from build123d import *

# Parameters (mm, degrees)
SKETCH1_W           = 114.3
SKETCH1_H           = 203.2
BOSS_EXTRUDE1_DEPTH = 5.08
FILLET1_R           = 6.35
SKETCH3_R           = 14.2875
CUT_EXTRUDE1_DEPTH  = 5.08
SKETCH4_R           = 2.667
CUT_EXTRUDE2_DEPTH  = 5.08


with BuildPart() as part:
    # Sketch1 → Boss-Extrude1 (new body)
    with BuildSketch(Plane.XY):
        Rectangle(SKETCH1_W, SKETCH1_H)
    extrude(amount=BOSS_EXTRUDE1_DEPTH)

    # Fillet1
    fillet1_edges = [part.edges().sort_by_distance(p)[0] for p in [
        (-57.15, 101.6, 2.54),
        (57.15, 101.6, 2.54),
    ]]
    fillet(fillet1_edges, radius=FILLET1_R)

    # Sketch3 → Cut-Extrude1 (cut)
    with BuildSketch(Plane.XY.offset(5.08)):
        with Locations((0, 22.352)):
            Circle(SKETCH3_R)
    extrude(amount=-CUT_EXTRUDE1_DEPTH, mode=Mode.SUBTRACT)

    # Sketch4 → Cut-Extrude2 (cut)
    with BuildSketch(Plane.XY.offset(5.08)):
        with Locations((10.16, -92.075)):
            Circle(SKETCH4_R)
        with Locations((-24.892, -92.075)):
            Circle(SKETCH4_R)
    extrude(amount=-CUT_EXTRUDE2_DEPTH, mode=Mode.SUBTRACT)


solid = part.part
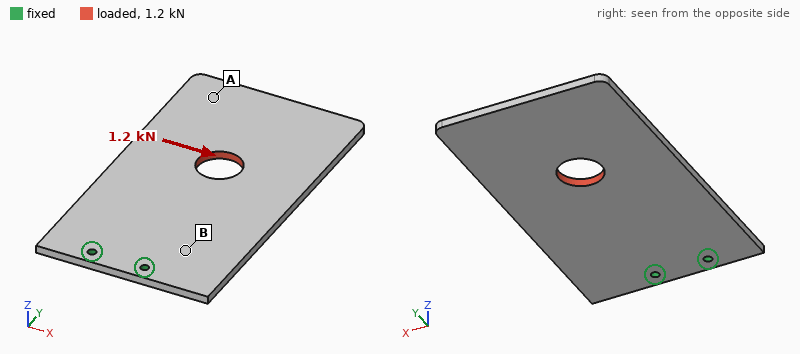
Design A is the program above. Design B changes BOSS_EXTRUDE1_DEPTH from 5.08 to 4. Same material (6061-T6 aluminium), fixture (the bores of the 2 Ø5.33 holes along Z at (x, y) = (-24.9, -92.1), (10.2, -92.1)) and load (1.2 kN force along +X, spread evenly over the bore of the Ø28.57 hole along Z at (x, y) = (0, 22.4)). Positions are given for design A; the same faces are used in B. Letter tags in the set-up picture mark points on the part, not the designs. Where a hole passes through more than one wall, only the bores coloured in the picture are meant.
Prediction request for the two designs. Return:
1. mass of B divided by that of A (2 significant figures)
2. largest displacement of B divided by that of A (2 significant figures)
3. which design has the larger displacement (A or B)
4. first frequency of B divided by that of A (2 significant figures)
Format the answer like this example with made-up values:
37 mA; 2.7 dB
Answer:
0.79; 1.3; B; 0.79
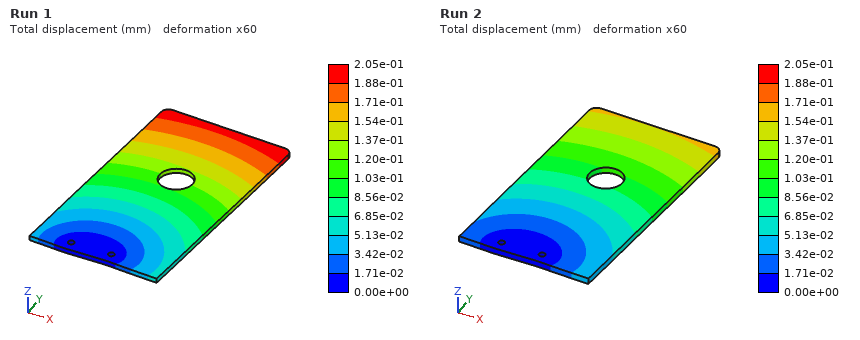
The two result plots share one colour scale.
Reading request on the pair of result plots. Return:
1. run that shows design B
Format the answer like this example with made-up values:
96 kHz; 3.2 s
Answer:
Run 1
